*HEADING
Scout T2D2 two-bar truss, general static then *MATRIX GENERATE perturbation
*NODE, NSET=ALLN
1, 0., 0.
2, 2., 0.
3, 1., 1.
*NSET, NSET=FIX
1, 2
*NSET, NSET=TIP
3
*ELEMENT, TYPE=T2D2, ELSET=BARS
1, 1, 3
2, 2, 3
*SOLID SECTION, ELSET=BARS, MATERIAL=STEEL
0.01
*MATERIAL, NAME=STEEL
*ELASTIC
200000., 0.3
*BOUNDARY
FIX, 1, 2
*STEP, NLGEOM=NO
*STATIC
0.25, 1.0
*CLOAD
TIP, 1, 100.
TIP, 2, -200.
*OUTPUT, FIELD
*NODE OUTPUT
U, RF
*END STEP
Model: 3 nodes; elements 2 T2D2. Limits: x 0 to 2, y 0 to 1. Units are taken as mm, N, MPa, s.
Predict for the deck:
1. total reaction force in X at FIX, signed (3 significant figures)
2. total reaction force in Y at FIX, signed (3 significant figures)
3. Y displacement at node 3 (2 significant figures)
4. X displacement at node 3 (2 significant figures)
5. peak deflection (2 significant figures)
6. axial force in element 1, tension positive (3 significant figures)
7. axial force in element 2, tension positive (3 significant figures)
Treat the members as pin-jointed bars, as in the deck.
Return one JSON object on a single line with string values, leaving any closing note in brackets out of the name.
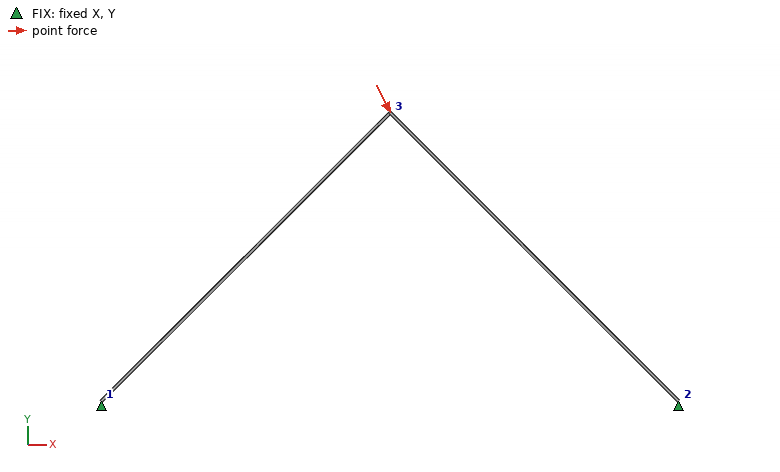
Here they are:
{"total reaction force in X at FIX, signed": "-100 N", "total reaction force in Y at FIX, signed": "200 N", "Y displacement at node 3": "-0.14 mm", "X displacement at node 3": "0.071 mm", "peak deflection": "0.16 mm", "axial force in element 1, tension positive": "-70.7 N", "axial force in element 2, tension positive": "-212 N"}
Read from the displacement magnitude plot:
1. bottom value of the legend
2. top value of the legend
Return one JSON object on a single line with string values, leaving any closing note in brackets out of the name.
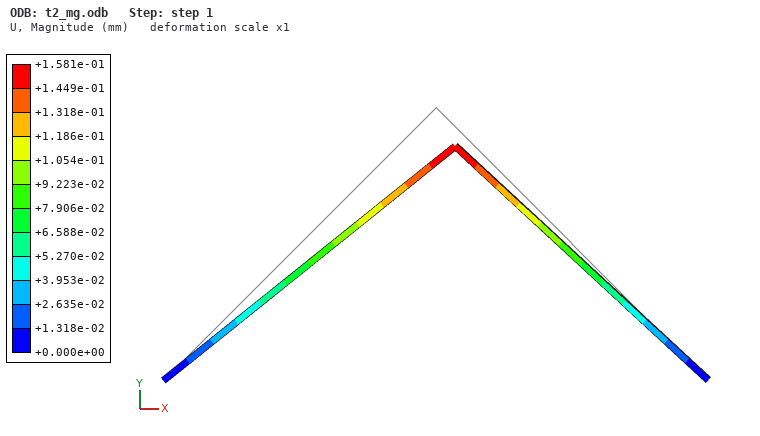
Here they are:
{"bottom value of the legend": "+0.000e+00 mm", "top value of the legend": "+1.581e-01 mm"}
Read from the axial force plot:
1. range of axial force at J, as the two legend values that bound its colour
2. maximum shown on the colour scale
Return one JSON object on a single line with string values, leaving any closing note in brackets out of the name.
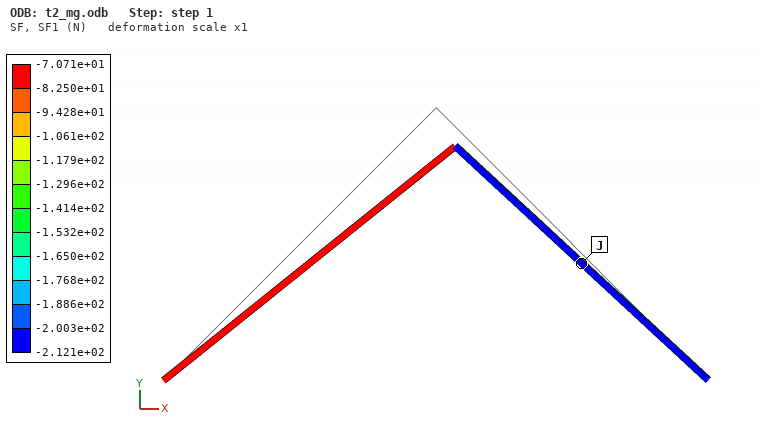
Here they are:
{"range of axial force at J, as the two legend values that bound its colour": "-2.121e+02 to -2.003e+02 N", "maximum shown on the colour scale": "-7.071e+01 N"}
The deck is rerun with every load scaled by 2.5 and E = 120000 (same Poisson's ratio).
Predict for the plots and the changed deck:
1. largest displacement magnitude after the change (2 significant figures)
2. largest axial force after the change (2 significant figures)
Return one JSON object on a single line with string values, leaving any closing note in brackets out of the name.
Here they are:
{"largest displacement magnitude after the change": "0.66 mm", "largest axial force after the change": "-180 N"}
